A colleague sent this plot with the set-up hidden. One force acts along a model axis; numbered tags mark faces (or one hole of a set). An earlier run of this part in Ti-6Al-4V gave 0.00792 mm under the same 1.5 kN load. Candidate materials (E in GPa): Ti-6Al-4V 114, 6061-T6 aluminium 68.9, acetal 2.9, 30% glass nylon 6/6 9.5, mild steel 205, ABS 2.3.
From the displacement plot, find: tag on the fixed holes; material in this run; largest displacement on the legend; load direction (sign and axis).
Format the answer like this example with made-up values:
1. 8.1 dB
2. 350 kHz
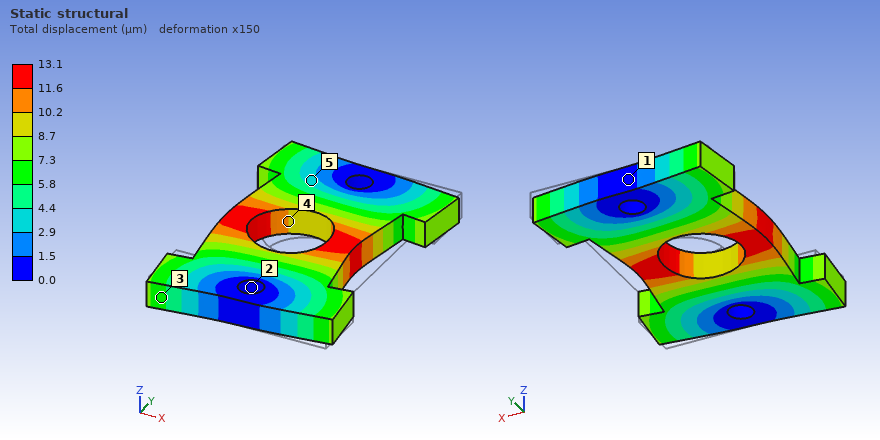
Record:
1. 2
2. 6061-T6 aluminium
3. 13.1 µm
4. -X
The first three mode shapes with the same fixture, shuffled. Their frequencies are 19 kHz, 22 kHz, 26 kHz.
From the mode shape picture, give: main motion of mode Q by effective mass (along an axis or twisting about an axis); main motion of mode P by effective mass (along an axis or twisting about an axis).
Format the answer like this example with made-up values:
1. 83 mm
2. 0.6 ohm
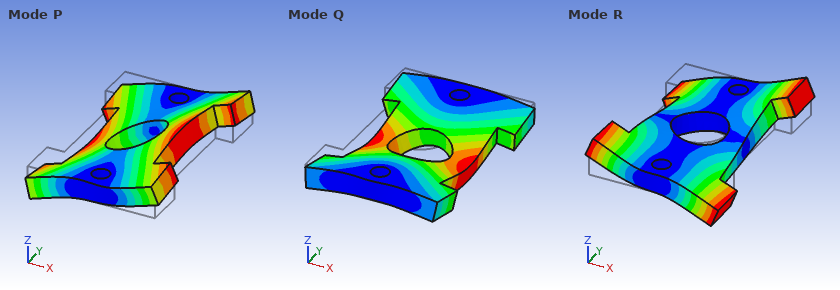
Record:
1. along Z
2. twisting about Y
